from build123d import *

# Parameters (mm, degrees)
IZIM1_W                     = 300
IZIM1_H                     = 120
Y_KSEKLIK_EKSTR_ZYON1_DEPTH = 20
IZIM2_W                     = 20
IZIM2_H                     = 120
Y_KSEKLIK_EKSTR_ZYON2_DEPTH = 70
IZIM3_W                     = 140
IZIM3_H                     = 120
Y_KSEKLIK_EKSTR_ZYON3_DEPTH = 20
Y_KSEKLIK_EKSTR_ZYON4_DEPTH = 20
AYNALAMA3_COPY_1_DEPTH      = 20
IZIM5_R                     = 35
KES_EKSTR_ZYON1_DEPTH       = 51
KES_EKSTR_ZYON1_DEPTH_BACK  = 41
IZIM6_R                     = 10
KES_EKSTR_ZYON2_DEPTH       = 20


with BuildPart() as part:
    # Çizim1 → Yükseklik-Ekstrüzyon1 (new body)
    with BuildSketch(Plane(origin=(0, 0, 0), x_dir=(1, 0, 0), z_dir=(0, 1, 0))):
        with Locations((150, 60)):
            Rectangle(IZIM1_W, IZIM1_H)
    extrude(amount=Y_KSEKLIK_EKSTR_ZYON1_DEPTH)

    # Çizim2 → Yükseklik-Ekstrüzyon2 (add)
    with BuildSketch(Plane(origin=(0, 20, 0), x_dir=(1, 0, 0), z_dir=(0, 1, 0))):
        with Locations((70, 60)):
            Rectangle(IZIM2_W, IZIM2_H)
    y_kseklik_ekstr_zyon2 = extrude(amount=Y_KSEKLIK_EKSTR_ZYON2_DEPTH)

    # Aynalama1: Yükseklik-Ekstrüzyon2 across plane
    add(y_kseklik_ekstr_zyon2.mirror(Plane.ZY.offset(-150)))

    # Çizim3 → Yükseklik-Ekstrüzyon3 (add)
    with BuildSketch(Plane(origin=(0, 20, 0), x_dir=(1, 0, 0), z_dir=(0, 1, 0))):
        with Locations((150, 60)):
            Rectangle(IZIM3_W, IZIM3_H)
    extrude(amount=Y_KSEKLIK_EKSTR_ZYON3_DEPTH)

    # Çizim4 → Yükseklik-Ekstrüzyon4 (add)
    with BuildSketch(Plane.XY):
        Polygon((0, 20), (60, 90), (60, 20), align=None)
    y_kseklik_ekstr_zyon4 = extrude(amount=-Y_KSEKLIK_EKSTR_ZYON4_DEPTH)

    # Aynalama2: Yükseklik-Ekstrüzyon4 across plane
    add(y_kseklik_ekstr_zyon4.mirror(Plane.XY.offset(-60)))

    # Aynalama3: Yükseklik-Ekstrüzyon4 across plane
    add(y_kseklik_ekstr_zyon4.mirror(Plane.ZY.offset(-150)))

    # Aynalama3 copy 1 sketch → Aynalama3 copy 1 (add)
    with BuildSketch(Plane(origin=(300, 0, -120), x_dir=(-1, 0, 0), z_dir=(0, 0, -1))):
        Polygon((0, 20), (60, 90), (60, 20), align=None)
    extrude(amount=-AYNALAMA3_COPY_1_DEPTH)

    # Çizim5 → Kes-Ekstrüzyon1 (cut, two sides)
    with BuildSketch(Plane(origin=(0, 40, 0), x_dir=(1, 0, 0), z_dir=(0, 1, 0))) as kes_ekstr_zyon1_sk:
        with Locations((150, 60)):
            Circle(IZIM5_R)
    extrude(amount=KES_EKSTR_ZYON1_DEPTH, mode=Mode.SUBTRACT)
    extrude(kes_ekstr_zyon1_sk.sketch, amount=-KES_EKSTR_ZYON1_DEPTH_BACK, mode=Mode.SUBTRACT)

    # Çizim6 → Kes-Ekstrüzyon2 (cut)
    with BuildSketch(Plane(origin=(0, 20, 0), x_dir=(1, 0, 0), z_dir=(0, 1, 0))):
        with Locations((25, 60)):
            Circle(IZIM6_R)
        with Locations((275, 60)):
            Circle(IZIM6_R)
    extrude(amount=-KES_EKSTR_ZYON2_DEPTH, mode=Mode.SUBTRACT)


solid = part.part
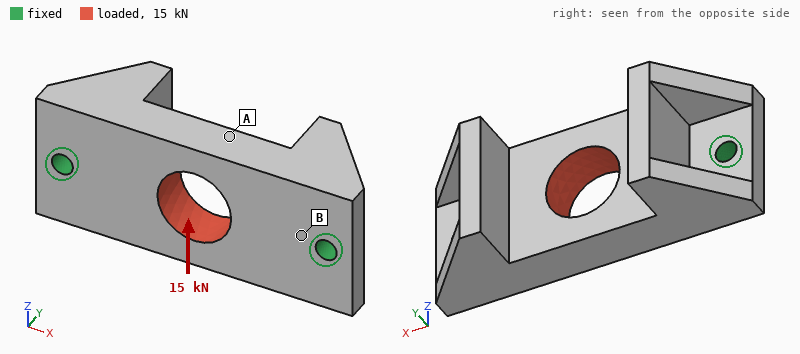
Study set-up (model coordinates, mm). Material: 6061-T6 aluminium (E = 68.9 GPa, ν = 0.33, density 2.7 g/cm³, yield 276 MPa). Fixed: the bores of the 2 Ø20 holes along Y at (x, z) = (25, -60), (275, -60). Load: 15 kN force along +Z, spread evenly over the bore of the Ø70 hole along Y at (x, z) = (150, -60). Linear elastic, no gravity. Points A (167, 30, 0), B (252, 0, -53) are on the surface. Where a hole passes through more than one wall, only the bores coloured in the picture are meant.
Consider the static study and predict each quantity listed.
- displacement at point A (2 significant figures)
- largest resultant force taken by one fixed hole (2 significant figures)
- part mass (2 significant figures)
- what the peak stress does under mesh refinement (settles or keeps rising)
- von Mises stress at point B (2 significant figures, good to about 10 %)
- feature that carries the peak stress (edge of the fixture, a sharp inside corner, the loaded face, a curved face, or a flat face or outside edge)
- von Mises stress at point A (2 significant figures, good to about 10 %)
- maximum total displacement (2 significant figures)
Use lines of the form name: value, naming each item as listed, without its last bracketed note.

displacement at point A: 33 µm
largest resultant force taken by one fixed hole: 7.5 kN
part mass: 3.8 kg
what the peak stress does under mesh refinement: keeps rising
von Mises stress at point B: 3.9 MPa
feature that carries the peak stress: edge of the fixture
von Mises stress at point A: 8.3 MPa
maximum total displacement: 41 µm
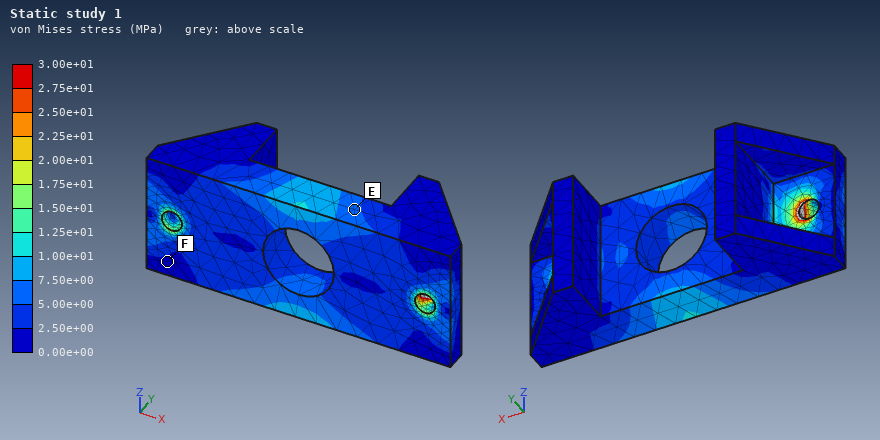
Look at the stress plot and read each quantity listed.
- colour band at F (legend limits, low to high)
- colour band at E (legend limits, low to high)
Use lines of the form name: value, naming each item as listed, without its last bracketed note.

colour band at F: 0.00e+00 to 2.50e+00 MPa
colour band at E: 5.00e+00 to 7.50e+00 MPa
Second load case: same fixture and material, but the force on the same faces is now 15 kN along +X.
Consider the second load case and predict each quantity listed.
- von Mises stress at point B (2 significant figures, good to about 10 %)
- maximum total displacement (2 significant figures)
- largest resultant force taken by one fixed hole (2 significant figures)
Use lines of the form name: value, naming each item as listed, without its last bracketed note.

von Mises stress at point B: 6.1 MPa
maximum total displacement: 6.6 µm
largest resultant force taken by one fixed hole: 7.5 kN
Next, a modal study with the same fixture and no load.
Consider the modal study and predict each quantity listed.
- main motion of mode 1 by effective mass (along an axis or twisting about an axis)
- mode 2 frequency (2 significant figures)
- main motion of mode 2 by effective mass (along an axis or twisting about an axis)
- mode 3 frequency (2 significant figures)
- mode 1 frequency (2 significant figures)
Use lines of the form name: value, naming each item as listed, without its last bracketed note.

main motion of mode 1 by effective mass: along Z
mode 2 frequency: 1600 Hz
main motion of mode 2 by effective mass: along Y
mode 3 frequency: 2500 Hz
mode 1 frequency: 1300 Hz
